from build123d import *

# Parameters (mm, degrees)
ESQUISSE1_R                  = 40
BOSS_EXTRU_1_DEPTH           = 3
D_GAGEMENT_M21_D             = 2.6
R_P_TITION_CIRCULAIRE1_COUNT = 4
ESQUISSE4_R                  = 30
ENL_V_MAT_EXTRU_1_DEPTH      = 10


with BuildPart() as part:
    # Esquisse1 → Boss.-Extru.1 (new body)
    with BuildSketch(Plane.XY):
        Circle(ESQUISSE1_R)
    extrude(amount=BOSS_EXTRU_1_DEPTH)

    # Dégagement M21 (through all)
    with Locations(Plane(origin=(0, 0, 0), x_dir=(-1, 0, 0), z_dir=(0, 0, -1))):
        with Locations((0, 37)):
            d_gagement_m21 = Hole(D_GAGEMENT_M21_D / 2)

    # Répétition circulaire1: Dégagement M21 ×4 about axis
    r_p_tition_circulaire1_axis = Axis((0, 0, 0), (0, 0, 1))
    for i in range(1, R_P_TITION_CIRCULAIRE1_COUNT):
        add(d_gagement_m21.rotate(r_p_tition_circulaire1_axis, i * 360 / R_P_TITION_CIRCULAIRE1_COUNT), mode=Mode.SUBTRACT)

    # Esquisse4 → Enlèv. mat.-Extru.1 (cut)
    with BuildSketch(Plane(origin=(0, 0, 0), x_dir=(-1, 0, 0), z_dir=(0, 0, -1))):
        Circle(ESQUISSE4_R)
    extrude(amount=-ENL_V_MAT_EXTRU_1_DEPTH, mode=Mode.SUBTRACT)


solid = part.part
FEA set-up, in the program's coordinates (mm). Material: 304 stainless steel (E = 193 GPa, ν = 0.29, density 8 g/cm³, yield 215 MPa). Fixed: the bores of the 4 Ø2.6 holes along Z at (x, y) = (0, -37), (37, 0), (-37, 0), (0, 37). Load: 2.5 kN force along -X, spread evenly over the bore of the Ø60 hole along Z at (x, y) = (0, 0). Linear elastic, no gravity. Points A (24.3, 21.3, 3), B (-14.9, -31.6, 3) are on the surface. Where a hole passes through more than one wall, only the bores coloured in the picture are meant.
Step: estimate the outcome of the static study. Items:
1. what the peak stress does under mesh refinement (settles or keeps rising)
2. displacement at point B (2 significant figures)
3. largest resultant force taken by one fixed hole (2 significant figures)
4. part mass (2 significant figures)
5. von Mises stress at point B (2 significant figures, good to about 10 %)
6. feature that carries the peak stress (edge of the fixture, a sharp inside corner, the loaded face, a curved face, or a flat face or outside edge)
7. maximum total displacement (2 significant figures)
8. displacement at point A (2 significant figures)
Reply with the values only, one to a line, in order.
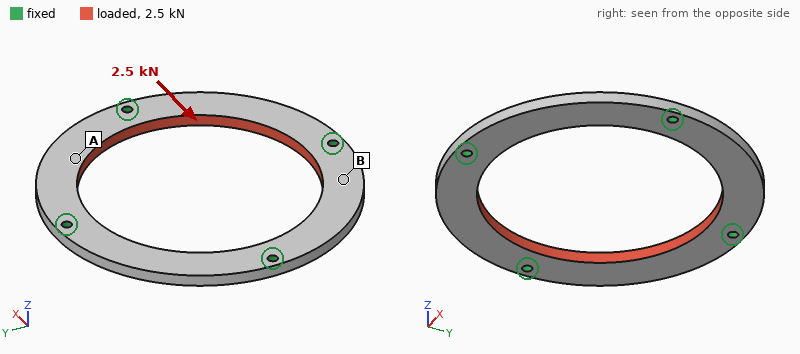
keeps rising
2.4 µm
890 N
52 g
11 MPa
edge of the fixture
3.5 µm
3.4 µm
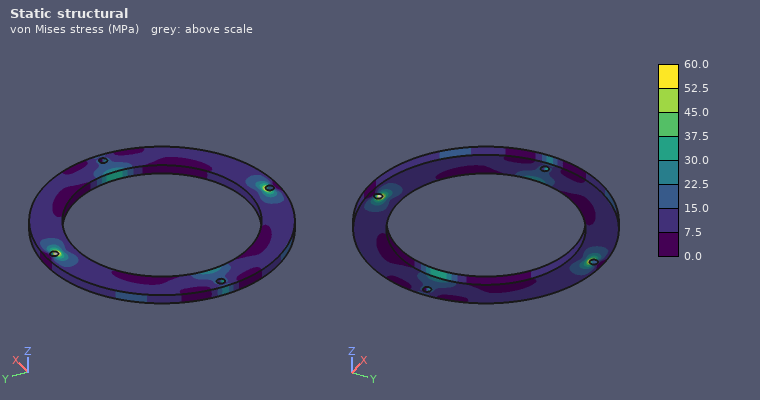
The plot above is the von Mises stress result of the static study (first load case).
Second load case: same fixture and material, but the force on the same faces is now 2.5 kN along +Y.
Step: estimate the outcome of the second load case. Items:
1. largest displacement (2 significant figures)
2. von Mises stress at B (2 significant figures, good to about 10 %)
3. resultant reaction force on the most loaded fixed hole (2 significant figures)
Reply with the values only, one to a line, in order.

3.5 µm
8.6 MPa
890 N
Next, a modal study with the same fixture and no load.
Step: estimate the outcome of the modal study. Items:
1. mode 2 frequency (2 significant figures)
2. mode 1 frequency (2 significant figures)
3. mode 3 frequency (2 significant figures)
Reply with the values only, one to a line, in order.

4500 Hz
4300 Hz
4500 Hz
